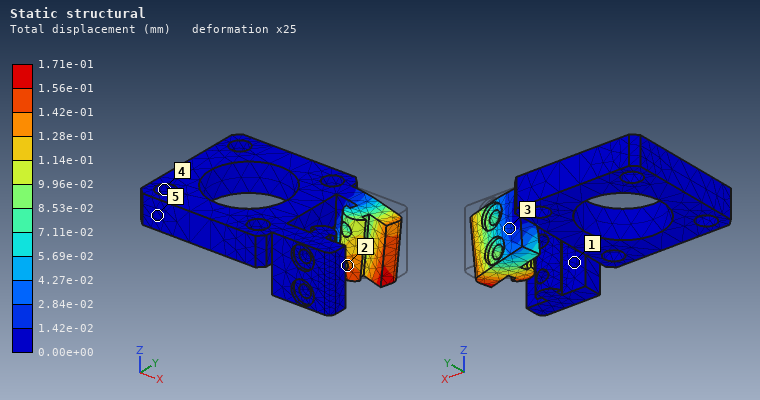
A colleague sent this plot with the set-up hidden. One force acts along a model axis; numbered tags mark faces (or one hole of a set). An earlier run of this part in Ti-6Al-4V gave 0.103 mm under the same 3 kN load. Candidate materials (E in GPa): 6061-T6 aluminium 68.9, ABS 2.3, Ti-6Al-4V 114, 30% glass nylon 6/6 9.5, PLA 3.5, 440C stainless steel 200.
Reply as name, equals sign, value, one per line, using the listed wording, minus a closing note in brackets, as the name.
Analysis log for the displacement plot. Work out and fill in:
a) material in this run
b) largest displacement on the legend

material in this run = 6061-T6 aluminium
largest displacement on the legend = 1.71e-01 mm
